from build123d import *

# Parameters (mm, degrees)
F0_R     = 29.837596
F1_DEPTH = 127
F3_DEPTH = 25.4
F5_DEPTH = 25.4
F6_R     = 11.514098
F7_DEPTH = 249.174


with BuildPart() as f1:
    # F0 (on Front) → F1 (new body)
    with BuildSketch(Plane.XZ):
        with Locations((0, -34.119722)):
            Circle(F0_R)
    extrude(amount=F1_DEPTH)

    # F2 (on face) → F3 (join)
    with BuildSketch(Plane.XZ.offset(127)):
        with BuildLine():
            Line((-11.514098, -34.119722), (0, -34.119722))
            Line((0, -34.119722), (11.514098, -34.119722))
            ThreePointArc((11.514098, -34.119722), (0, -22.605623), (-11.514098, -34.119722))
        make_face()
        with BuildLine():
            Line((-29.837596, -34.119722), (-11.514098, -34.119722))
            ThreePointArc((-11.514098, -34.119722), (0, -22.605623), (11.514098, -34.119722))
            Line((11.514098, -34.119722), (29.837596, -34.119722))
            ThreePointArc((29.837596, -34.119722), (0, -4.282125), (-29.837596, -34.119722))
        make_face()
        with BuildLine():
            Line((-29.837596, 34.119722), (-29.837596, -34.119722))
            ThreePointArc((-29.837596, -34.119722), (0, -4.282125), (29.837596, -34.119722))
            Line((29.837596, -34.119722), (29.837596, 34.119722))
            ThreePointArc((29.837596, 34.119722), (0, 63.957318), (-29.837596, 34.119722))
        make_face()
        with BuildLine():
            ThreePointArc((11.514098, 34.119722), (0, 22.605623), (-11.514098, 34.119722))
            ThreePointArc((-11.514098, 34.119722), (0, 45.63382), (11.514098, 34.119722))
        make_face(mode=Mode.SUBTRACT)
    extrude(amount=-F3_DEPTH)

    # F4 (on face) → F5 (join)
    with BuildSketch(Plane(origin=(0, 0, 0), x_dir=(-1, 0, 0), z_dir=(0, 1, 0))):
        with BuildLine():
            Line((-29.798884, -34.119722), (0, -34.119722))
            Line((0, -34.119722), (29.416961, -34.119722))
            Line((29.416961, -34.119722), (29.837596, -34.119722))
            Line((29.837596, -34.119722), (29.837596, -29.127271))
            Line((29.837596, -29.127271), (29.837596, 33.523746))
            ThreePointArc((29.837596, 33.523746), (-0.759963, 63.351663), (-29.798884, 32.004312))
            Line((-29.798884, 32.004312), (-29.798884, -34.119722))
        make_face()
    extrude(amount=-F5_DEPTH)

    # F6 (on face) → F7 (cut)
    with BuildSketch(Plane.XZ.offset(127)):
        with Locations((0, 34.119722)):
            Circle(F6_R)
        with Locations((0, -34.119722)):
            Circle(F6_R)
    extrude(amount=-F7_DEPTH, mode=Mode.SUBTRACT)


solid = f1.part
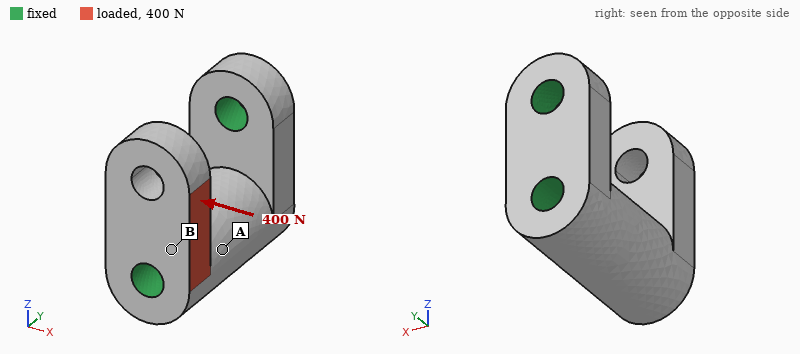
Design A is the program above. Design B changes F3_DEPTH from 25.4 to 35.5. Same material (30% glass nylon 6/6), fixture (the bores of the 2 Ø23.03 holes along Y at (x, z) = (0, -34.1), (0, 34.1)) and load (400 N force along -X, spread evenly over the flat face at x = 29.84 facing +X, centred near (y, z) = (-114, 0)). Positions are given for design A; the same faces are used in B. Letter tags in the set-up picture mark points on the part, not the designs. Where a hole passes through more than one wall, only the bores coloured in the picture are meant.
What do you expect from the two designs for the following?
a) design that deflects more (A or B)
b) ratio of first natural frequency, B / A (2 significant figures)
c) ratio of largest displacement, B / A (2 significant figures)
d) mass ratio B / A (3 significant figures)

A
1.2
0.77
1.08
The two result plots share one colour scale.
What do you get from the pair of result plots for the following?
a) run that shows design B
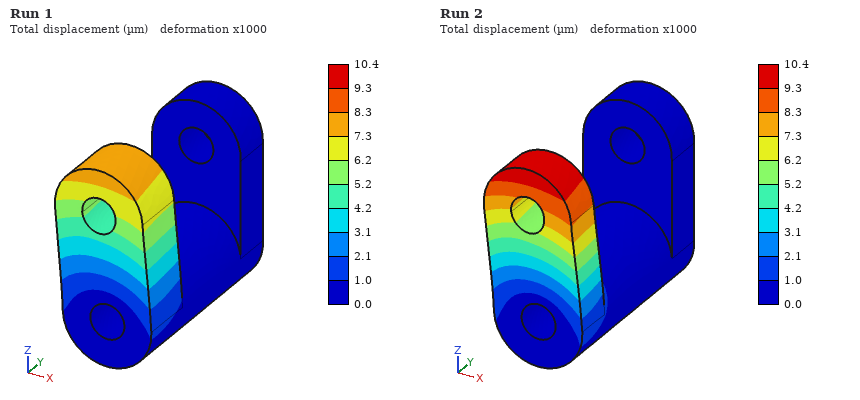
Run 1
